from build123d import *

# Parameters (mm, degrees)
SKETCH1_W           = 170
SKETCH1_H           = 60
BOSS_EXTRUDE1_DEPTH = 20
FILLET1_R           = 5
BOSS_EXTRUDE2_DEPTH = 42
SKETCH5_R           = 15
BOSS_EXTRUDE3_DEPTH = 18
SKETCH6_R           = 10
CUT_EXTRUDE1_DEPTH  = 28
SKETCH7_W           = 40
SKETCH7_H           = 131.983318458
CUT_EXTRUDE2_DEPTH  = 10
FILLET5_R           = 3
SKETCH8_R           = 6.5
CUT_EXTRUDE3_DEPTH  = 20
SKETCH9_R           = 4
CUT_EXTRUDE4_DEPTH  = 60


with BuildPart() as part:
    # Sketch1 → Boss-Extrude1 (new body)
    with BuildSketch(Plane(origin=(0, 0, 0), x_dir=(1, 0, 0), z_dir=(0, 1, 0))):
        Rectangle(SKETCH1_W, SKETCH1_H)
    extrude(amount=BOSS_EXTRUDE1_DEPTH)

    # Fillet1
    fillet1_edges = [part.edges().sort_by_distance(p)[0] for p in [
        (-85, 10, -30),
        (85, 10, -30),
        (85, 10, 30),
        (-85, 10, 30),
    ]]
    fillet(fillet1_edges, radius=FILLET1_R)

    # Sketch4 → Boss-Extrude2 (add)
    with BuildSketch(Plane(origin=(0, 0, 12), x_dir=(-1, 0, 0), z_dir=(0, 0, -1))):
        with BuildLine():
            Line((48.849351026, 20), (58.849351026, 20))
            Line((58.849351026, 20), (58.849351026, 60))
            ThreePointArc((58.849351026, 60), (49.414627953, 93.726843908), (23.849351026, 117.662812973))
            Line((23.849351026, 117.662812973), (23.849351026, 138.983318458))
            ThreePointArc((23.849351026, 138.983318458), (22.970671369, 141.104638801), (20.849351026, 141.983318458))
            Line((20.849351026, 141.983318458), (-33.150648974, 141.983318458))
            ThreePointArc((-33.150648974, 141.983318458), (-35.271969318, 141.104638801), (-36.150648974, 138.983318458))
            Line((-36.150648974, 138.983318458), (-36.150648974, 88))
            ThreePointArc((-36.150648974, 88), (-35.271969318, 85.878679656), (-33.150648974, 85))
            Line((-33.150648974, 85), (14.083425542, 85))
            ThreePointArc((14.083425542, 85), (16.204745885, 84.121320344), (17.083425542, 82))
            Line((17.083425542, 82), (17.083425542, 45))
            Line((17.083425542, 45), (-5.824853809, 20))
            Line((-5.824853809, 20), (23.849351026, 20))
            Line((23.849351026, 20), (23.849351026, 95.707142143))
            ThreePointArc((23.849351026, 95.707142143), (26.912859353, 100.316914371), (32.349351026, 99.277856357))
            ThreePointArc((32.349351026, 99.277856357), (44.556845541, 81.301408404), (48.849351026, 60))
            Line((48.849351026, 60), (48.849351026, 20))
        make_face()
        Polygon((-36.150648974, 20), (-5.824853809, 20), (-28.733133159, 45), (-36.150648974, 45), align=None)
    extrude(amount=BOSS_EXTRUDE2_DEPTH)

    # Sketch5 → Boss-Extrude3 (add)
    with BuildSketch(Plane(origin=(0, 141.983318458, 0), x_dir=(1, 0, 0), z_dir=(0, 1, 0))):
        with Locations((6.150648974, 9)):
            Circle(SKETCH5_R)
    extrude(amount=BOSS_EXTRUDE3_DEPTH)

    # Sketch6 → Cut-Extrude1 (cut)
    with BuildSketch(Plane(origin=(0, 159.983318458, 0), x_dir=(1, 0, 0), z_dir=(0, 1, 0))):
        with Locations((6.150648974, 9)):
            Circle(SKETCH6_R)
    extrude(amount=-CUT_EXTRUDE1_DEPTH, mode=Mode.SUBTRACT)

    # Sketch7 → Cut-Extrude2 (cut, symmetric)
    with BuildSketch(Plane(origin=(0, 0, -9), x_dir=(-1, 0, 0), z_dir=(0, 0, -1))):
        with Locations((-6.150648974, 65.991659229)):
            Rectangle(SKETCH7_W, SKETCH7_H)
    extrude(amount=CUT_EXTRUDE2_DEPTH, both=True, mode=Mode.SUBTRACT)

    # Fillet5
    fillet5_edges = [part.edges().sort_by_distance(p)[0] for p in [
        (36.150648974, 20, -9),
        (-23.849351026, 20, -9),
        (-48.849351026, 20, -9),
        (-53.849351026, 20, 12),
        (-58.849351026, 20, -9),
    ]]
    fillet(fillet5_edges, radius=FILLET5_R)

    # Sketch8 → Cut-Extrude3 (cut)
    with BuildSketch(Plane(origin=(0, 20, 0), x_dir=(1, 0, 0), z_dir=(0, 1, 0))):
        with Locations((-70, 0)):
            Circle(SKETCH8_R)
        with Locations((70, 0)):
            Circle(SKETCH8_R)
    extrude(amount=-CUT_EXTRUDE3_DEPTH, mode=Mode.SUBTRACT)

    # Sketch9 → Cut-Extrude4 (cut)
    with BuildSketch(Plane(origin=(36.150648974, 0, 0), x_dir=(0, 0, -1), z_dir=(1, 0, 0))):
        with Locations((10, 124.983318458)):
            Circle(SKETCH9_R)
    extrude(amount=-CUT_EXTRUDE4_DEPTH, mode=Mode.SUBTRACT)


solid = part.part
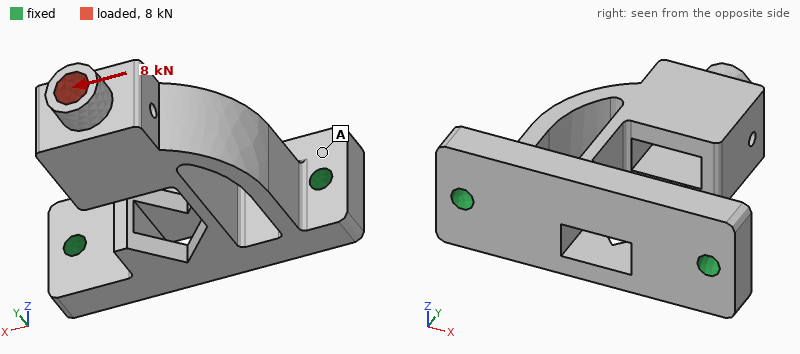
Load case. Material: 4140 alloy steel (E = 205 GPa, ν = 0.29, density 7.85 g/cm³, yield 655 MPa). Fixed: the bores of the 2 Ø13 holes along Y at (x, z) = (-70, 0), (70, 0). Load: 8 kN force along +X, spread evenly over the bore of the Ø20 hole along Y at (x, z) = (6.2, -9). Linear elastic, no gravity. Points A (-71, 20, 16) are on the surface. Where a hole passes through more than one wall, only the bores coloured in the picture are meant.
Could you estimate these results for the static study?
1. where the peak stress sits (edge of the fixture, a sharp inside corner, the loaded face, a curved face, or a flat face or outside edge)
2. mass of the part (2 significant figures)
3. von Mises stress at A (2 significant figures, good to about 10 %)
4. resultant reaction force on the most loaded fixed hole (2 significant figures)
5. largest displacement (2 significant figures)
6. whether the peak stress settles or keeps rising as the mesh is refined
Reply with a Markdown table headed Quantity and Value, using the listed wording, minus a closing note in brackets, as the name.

| Quantity | Value |
|---|---|
| where the peak stress sits | a sharp inside corner |
| mass of the part | 3.0 kg |
| von Mises stress at A | 30 MPa |
| resultant reaction force on the most loaded fixed hole | 8.9 kN |
| largest displacement | 0.60 mm |
| whether the peak stress settles or keeps rising as the mesh is refined | keeps rising |
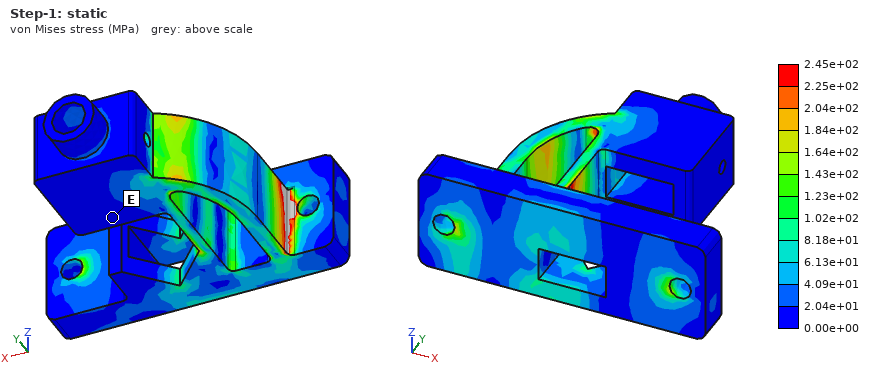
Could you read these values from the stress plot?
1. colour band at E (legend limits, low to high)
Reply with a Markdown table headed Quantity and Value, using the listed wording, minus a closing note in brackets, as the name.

| Quantity | Value |
|---|---|
| colour band at E | 0.00e+00 to 2.04e+01 MPa |
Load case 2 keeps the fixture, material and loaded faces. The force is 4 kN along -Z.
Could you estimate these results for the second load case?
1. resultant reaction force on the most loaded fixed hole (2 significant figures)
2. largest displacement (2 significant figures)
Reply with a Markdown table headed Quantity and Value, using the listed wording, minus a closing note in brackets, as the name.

| Quantity | Value |
|---|---|
| resultant reaction force on the most loaded fixed hole | 2.1 kN |
| largest displacement | 0.50 mm |
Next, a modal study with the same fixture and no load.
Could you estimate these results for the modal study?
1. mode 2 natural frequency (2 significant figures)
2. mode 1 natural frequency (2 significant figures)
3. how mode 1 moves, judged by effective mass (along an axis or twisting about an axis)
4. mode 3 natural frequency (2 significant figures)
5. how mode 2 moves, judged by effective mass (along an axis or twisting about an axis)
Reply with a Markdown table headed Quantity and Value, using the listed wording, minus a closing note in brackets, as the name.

| Quantity | Value |
|---|---|
| mode 2 natural frequency | 770 Hz |
| mode 1 natural frequency | 610 Hz |
| how mode 1 moves, judged by effective mass | along Z |
| mode 3 natural frequency | 1400 Hz |
| how mode 2 moves, judged by effective mass | along X |
